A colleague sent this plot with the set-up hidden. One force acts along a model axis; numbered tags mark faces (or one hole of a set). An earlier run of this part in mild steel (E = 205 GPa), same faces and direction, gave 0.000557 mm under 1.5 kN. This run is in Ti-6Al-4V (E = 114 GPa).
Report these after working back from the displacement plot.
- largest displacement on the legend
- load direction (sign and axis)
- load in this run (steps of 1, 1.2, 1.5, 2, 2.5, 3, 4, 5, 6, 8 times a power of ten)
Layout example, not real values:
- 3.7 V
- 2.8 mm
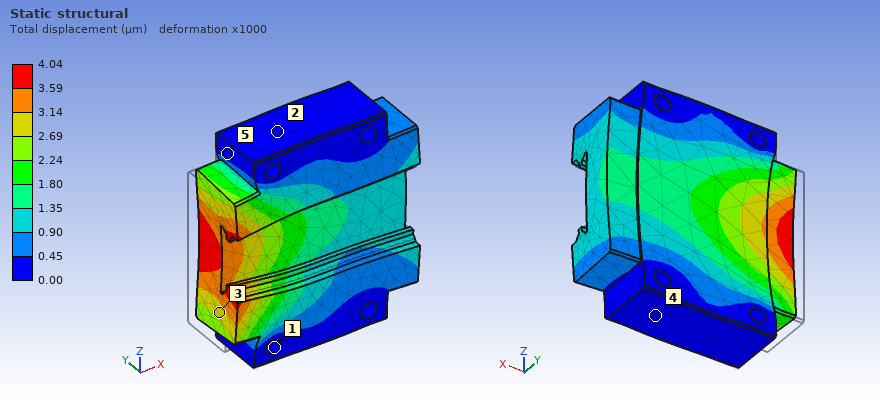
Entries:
- 4.04 µm
- +X
- 6 kN
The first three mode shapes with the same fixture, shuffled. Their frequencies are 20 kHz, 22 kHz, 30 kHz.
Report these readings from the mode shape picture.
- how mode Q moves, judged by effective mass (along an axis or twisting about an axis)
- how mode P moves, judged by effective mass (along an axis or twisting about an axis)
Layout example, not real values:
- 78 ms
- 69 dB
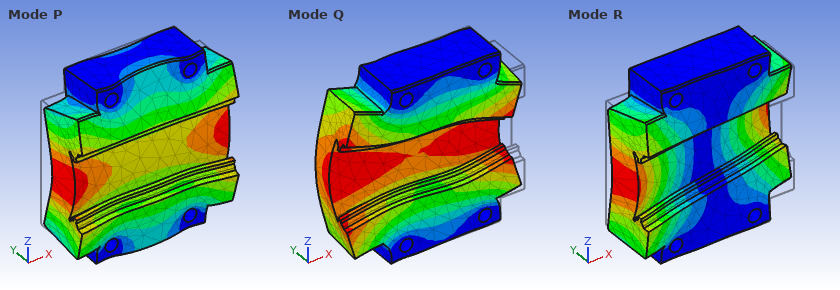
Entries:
- along X
- along Y
